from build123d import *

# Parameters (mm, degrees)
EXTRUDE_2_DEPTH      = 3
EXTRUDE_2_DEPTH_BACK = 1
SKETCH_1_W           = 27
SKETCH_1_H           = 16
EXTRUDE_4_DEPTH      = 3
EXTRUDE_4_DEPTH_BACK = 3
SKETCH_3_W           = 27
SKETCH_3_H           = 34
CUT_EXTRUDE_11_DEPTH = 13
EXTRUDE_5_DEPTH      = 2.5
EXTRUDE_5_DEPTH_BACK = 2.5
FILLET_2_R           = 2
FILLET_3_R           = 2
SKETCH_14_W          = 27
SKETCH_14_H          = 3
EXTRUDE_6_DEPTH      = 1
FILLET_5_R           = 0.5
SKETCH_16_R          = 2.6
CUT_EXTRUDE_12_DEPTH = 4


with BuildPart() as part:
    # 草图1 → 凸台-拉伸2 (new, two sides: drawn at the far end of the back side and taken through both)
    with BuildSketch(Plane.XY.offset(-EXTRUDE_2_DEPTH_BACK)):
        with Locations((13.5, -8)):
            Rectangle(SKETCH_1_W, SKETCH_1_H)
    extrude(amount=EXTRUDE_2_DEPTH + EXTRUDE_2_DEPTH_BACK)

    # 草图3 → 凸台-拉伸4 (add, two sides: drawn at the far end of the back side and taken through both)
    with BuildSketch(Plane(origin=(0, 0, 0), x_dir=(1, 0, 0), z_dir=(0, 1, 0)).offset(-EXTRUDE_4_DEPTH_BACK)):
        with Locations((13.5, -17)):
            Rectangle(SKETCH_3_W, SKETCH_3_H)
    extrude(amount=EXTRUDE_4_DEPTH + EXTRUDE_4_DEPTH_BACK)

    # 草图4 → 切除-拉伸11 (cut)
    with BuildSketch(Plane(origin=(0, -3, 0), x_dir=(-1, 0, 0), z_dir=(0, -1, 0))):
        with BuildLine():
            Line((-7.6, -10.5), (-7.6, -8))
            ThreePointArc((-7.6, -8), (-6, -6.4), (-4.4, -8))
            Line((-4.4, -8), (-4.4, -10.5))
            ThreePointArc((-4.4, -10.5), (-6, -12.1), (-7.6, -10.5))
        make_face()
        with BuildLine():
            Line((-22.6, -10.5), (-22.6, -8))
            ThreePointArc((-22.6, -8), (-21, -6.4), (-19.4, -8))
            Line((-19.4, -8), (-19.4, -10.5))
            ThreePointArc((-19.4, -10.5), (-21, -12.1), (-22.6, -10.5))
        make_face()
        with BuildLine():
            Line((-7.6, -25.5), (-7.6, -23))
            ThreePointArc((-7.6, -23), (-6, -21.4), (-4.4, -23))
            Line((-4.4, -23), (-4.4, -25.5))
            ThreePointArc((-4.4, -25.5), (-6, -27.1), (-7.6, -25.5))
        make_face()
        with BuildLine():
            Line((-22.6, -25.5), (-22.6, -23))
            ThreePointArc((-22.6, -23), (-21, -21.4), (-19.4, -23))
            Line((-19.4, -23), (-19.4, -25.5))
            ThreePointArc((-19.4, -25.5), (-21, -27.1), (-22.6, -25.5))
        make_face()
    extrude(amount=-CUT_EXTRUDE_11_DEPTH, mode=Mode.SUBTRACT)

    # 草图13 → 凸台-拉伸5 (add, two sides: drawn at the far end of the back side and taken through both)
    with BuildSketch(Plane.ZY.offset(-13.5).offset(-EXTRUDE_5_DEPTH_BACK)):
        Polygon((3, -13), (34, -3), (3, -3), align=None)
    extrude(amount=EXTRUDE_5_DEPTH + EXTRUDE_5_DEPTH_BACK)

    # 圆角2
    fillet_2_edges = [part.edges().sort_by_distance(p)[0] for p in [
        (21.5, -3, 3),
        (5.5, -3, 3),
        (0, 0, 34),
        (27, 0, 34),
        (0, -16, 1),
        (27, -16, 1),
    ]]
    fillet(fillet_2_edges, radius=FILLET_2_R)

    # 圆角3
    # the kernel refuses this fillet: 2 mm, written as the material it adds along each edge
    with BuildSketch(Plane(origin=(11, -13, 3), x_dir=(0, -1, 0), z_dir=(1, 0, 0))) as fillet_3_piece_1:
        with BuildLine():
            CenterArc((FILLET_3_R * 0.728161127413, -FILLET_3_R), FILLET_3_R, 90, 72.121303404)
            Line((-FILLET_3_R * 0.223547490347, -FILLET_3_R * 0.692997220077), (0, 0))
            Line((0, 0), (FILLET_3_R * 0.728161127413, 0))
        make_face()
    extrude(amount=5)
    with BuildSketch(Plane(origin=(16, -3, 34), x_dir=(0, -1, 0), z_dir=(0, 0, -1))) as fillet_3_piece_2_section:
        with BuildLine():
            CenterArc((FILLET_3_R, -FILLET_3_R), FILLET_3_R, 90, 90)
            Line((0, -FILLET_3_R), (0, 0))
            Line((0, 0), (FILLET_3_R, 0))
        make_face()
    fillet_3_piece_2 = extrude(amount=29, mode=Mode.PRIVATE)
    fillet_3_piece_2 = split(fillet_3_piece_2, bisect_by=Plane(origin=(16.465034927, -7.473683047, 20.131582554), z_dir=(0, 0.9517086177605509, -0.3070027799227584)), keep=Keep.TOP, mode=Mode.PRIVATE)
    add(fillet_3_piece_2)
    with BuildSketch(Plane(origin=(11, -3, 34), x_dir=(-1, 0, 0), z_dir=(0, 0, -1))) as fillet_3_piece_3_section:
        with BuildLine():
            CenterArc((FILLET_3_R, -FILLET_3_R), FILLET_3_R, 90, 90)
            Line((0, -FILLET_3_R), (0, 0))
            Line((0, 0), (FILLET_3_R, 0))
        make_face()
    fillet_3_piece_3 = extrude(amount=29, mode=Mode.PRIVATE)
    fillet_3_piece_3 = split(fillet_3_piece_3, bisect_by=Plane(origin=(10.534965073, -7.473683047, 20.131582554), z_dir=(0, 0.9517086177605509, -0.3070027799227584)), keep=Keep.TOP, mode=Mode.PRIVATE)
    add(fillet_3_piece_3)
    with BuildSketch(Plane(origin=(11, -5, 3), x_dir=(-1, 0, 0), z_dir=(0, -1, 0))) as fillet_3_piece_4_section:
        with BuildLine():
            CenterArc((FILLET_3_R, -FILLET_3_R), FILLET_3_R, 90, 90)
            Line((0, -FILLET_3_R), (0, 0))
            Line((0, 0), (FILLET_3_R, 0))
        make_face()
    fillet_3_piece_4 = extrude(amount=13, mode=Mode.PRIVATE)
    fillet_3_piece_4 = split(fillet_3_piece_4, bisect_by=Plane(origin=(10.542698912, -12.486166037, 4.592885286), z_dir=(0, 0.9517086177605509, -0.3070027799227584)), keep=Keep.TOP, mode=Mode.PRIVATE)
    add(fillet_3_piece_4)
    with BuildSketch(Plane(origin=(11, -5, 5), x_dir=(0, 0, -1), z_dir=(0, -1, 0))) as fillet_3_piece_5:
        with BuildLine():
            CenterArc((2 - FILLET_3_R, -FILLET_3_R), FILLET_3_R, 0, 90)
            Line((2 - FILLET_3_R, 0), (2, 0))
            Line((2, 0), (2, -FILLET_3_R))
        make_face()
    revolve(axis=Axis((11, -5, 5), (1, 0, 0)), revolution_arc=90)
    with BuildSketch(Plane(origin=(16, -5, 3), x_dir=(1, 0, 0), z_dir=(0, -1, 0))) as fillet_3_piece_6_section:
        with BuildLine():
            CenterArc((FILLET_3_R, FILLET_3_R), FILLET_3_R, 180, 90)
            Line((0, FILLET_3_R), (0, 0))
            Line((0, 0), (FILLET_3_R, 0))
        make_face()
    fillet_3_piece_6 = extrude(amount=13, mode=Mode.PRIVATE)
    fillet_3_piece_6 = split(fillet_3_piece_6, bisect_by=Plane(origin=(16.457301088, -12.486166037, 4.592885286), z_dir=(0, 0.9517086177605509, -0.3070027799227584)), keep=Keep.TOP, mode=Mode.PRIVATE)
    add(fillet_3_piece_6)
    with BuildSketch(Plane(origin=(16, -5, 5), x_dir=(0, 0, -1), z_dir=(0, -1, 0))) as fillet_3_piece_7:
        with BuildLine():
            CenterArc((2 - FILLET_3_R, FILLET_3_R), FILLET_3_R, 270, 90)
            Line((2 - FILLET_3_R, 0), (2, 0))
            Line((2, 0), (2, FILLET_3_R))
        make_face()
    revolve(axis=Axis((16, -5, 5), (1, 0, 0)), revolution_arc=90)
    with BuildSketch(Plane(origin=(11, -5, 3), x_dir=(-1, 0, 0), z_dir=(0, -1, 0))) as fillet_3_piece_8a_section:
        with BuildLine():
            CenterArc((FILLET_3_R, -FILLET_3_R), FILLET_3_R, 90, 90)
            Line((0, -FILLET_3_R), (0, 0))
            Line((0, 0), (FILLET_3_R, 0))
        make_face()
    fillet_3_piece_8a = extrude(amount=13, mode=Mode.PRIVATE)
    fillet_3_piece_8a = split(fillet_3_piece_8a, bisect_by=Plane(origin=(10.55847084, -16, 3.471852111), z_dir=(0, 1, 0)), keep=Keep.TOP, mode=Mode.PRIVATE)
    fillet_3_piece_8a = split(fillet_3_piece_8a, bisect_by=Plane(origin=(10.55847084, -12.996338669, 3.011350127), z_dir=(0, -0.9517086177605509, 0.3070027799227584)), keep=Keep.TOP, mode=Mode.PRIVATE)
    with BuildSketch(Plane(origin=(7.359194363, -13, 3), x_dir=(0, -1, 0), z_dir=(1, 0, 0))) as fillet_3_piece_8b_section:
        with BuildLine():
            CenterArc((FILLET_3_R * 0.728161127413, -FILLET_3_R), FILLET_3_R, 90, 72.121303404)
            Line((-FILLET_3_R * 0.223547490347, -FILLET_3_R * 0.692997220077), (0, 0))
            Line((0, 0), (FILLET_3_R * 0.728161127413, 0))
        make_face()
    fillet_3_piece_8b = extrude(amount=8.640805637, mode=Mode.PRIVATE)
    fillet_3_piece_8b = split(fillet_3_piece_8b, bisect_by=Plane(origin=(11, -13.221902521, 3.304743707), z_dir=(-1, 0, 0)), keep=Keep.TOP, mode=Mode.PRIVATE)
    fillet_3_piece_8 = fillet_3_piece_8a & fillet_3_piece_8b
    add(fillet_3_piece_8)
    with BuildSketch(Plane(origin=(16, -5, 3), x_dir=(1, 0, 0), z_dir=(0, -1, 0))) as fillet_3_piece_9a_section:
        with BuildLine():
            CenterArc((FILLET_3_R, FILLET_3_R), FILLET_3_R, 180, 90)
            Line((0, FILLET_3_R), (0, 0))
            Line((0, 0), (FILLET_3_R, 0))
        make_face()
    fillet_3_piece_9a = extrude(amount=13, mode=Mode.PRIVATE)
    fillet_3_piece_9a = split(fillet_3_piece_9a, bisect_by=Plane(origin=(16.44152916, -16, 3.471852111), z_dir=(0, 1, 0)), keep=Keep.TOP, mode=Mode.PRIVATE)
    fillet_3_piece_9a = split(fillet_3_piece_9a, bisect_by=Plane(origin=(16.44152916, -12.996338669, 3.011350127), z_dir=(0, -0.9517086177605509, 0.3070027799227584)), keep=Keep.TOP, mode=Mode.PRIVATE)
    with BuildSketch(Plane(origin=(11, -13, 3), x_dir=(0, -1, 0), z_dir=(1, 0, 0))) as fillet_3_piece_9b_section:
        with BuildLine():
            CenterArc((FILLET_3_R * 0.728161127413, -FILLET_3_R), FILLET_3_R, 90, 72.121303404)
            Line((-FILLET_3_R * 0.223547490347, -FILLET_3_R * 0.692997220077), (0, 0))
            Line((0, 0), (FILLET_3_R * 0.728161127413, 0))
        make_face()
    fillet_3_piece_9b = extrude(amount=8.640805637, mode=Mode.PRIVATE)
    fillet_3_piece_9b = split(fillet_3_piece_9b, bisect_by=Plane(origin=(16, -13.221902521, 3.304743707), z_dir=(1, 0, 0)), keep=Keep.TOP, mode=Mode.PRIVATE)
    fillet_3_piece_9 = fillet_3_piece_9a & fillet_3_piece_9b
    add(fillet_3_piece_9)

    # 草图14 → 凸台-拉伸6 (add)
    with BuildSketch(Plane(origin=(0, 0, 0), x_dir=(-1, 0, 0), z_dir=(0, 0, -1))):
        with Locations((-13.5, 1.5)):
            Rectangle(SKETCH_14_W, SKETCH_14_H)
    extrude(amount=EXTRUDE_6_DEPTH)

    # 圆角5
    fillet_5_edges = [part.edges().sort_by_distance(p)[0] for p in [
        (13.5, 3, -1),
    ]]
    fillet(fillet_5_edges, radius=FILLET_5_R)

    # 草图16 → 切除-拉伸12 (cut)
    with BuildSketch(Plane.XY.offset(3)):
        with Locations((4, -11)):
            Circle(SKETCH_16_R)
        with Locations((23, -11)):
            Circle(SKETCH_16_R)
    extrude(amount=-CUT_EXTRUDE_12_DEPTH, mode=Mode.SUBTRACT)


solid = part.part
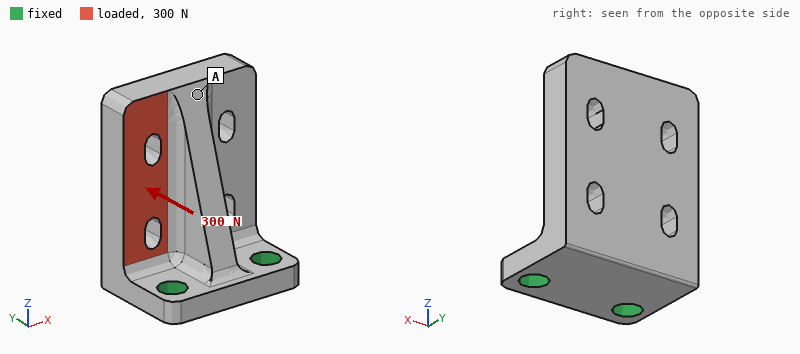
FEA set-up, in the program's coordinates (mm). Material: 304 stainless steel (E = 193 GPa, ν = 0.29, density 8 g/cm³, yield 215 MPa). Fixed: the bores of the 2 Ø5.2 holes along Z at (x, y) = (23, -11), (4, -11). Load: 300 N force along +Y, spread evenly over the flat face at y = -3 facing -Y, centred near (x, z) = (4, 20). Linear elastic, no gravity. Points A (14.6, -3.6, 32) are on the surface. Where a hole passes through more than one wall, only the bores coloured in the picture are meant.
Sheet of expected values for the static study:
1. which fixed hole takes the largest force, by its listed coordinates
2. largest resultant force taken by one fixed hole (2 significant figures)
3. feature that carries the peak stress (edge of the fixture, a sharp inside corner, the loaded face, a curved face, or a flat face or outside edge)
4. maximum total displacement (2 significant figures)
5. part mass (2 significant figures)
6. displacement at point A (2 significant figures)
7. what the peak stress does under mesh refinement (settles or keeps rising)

(4, -11)
290 N
a sharp inside corner
29 µm
59 g
22 µm
keeps rising
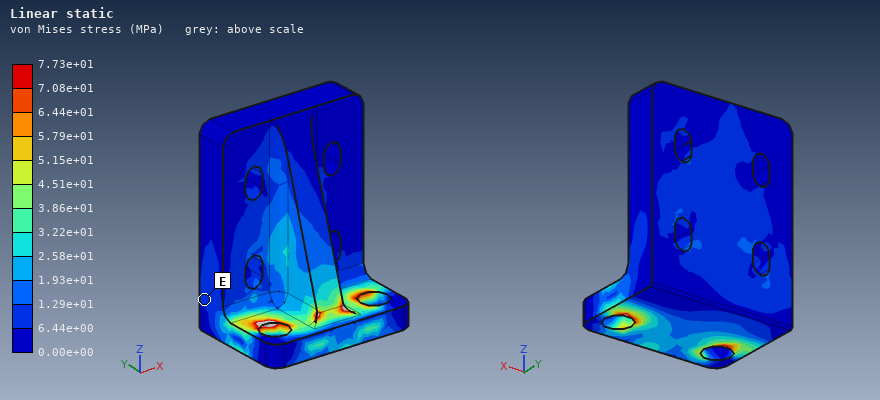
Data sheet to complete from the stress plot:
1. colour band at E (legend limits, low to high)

6.44e+00 to 1.29e+01 MPa
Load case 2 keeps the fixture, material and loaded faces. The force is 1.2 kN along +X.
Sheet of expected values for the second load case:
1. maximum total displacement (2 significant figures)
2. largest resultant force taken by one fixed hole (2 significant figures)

35 µm
1.5 kN
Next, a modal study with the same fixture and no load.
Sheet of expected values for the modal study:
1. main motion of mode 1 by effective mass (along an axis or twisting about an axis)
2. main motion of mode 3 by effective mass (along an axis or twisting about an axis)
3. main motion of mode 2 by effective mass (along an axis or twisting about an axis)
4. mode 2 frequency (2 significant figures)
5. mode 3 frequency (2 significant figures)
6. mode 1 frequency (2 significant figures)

along Y
twisting about Z
along X
5900 Hz
11 kHz
3300 Hz
